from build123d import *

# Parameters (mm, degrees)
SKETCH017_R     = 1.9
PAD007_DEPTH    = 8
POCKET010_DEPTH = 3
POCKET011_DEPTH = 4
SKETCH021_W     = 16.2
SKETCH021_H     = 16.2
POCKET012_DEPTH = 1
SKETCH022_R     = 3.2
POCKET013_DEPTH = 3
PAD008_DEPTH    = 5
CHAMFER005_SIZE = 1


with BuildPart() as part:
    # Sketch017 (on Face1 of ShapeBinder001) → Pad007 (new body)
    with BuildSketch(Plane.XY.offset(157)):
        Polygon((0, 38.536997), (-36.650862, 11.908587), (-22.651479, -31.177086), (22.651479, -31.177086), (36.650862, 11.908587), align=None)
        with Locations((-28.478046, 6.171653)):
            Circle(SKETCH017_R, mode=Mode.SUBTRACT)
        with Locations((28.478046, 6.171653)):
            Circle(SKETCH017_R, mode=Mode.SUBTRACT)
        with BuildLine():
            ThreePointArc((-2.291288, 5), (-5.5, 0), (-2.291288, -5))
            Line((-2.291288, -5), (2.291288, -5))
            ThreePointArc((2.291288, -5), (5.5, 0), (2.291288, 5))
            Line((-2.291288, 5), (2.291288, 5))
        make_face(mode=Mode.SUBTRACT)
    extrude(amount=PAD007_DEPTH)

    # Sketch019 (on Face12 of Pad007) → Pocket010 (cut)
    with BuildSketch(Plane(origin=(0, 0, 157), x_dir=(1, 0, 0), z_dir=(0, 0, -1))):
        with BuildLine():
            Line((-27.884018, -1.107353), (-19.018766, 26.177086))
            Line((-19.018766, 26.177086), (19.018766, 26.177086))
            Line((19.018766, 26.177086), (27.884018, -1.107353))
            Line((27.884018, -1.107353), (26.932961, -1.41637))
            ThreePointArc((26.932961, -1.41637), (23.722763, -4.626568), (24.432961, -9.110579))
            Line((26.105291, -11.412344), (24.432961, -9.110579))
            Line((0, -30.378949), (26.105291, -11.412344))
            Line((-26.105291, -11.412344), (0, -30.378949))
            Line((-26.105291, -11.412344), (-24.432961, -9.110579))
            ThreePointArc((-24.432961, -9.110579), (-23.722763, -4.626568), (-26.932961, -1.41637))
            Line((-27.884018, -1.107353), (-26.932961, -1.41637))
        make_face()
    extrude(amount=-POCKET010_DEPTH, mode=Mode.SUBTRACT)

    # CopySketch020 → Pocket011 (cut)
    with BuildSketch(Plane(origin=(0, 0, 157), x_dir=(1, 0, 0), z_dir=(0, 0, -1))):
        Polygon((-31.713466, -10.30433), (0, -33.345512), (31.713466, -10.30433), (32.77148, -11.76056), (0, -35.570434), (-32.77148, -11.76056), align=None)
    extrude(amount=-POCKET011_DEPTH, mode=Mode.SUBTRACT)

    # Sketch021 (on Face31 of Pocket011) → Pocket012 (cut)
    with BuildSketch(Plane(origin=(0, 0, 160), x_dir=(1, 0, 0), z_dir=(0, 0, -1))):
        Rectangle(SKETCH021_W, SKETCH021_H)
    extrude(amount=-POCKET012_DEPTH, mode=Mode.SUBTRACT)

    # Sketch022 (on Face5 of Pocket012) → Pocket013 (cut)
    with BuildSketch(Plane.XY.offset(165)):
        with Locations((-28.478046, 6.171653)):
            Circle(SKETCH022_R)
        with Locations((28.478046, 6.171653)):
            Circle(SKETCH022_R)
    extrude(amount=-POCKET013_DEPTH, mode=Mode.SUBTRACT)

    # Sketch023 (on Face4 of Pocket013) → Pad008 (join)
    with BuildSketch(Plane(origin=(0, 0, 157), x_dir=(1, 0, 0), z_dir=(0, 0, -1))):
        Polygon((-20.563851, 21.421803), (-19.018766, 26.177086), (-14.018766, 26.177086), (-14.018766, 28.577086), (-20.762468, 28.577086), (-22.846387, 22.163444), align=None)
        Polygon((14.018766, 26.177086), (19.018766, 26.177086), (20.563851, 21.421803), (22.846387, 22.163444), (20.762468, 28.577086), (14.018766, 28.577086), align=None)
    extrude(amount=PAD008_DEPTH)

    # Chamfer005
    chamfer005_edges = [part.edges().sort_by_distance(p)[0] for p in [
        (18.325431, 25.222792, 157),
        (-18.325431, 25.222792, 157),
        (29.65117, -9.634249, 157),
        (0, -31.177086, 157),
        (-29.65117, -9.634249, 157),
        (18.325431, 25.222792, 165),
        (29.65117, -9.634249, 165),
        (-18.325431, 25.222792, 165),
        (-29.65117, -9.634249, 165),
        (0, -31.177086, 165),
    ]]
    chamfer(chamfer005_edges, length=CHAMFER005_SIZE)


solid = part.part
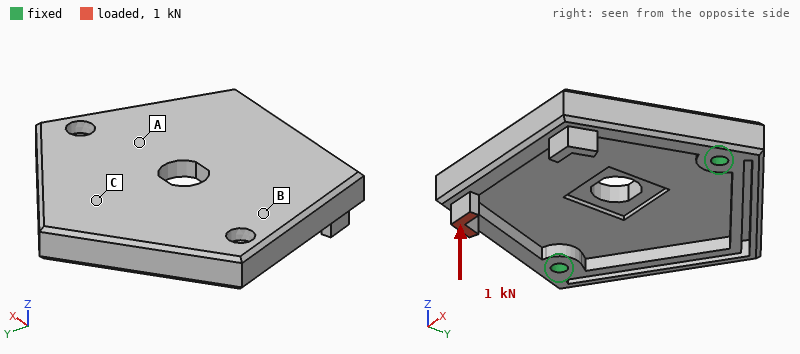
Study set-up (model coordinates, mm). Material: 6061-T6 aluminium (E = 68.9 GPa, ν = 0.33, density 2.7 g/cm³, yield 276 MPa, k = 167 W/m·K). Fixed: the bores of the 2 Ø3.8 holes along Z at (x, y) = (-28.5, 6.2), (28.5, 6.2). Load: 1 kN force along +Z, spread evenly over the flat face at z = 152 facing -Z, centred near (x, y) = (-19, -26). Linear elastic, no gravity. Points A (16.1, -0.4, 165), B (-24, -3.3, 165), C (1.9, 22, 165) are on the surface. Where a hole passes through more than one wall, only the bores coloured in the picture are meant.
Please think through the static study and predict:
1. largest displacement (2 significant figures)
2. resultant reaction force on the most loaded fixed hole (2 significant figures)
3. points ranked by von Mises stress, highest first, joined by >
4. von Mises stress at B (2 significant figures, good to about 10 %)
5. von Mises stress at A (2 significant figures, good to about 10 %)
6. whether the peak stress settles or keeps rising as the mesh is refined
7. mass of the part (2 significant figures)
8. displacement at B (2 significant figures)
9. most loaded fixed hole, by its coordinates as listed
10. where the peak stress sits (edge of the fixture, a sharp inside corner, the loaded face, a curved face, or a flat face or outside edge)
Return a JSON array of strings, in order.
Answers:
["0.45 mm", "1.0 kN", "B > A > C", "94 MPa", "48 MPa", "keeps rising", "54 g", "0.078 mm", "(-28.5, 6.2)", "edge of the fixture"]
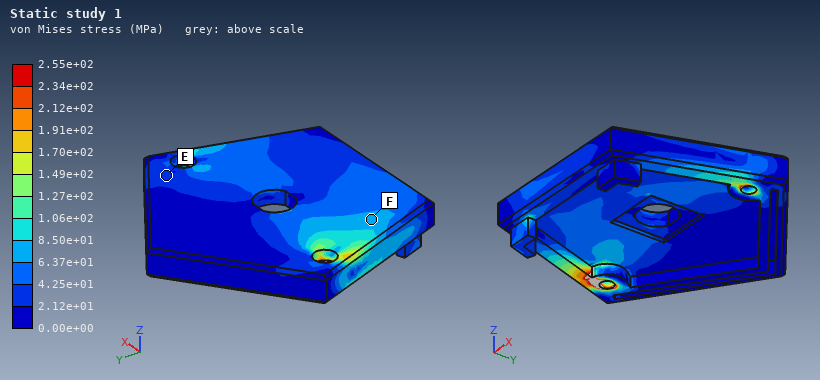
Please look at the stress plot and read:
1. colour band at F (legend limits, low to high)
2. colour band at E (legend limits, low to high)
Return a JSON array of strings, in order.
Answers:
["6.37e+01 to 8.50e+01 MPa", "2.12e+01 to 4.25e+01 MPa"]
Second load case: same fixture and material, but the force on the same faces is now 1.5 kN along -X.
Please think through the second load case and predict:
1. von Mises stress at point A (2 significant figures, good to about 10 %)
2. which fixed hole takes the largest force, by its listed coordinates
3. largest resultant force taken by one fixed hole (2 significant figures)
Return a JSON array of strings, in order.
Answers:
["16 MPa", "(-28.5, 6.2)", "1.3 kN"]
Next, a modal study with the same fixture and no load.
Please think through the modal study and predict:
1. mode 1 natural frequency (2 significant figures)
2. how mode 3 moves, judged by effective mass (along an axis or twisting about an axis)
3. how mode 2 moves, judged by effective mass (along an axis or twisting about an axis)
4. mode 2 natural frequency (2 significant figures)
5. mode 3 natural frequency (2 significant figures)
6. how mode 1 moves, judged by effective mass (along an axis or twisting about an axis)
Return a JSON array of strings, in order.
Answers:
["2400 Hz", "twisting about Y", "along Z", "4500 Hz", "5800 Hz", "along Z"]
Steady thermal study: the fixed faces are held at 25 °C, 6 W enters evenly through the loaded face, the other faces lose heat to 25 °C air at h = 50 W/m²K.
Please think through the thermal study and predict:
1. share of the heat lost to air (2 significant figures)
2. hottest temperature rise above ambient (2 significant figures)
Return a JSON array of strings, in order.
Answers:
["17 %", "15 K"]
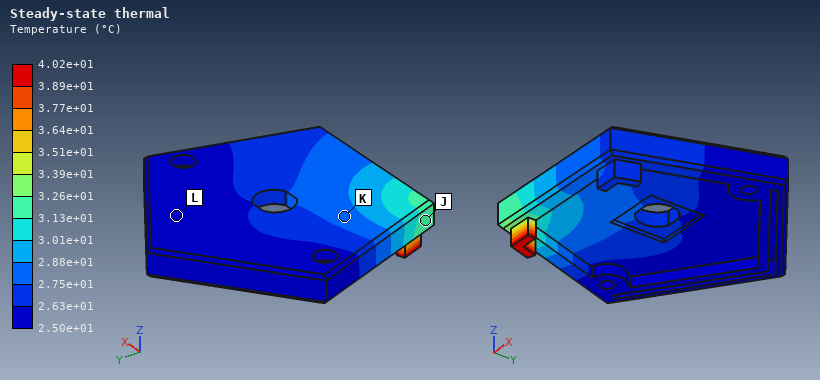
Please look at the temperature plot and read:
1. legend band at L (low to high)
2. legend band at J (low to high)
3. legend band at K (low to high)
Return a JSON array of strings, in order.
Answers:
["2.50e+01 to 2.63e+01 °C", "3.13e+01 to 3.26e+01 °C", "2.75e+01 to 2.88e+01 °C"]
